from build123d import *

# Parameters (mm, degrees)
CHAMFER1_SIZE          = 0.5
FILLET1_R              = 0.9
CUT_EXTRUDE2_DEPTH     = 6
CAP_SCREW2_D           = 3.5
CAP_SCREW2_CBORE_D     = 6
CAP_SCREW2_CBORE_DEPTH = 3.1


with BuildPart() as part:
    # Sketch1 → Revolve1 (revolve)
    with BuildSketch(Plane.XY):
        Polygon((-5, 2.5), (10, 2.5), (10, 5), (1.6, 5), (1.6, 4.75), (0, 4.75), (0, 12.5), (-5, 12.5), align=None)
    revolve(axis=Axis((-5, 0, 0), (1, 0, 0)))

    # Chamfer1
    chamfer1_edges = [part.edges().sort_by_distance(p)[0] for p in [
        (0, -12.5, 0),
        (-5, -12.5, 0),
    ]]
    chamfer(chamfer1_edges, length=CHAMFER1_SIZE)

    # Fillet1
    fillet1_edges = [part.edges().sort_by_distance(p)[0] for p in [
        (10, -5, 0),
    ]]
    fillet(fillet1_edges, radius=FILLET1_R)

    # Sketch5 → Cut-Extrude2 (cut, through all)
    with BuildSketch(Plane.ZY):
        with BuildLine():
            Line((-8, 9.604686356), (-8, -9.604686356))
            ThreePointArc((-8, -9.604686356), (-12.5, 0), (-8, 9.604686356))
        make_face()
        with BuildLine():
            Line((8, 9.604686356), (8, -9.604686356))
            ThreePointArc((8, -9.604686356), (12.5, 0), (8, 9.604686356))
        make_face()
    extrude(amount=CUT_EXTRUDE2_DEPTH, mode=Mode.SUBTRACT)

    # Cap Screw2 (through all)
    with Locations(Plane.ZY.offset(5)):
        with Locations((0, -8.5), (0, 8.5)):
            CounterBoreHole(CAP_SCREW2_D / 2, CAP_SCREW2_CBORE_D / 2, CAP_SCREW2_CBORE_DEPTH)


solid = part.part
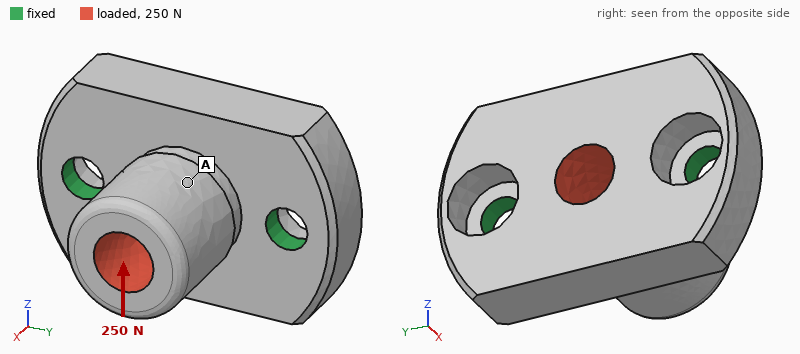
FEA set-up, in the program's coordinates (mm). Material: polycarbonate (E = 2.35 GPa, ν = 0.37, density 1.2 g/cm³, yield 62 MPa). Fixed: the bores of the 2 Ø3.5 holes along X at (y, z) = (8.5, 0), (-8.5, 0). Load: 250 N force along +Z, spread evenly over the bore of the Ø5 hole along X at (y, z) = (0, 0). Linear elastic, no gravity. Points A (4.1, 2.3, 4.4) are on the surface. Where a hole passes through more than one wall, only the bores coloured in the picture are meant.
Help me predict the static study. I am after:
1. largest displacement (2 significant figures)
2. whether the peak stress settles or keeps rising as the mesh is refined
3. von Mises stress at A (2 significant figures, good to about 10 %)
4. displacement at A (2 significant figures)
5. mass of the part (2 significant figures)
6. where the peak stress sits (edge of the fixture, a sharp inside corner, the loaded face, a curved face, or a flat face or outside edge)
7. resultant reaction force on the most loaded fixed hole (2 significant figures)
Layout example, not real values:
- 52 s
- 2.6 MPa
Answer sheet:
- 0.28 mm
- keeps rising
- 3.2 MPa
- 0.16 mm
- 2.5 g
- edge of the fixture
- 130 N
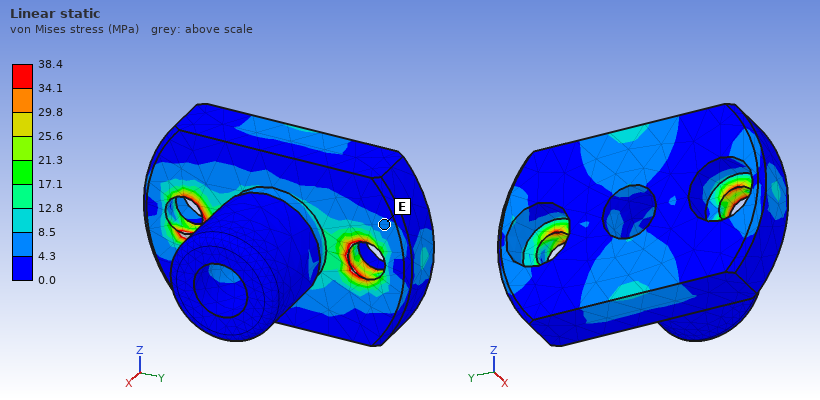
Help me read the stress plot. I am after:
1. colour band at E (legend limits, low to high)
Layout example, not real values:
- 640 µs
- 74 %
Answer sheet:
- 4.3 to 8.5 MPa
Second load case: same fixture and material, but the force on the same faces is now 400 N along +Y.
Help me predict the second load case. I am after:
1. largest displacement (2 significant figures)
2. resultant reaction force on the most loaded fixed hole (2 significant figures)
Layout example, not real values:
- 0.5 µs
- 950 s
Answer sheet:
- 0.18 mm
- 220 N
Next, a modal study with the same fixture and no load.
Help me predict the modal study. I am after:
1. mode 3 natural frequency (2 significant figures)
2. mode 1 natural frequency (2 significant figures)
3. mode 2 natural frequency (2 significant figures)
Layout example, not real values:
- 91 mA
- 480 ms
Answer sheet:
- 8700 Hz
- 4000 Hz
- 8600 Hz
